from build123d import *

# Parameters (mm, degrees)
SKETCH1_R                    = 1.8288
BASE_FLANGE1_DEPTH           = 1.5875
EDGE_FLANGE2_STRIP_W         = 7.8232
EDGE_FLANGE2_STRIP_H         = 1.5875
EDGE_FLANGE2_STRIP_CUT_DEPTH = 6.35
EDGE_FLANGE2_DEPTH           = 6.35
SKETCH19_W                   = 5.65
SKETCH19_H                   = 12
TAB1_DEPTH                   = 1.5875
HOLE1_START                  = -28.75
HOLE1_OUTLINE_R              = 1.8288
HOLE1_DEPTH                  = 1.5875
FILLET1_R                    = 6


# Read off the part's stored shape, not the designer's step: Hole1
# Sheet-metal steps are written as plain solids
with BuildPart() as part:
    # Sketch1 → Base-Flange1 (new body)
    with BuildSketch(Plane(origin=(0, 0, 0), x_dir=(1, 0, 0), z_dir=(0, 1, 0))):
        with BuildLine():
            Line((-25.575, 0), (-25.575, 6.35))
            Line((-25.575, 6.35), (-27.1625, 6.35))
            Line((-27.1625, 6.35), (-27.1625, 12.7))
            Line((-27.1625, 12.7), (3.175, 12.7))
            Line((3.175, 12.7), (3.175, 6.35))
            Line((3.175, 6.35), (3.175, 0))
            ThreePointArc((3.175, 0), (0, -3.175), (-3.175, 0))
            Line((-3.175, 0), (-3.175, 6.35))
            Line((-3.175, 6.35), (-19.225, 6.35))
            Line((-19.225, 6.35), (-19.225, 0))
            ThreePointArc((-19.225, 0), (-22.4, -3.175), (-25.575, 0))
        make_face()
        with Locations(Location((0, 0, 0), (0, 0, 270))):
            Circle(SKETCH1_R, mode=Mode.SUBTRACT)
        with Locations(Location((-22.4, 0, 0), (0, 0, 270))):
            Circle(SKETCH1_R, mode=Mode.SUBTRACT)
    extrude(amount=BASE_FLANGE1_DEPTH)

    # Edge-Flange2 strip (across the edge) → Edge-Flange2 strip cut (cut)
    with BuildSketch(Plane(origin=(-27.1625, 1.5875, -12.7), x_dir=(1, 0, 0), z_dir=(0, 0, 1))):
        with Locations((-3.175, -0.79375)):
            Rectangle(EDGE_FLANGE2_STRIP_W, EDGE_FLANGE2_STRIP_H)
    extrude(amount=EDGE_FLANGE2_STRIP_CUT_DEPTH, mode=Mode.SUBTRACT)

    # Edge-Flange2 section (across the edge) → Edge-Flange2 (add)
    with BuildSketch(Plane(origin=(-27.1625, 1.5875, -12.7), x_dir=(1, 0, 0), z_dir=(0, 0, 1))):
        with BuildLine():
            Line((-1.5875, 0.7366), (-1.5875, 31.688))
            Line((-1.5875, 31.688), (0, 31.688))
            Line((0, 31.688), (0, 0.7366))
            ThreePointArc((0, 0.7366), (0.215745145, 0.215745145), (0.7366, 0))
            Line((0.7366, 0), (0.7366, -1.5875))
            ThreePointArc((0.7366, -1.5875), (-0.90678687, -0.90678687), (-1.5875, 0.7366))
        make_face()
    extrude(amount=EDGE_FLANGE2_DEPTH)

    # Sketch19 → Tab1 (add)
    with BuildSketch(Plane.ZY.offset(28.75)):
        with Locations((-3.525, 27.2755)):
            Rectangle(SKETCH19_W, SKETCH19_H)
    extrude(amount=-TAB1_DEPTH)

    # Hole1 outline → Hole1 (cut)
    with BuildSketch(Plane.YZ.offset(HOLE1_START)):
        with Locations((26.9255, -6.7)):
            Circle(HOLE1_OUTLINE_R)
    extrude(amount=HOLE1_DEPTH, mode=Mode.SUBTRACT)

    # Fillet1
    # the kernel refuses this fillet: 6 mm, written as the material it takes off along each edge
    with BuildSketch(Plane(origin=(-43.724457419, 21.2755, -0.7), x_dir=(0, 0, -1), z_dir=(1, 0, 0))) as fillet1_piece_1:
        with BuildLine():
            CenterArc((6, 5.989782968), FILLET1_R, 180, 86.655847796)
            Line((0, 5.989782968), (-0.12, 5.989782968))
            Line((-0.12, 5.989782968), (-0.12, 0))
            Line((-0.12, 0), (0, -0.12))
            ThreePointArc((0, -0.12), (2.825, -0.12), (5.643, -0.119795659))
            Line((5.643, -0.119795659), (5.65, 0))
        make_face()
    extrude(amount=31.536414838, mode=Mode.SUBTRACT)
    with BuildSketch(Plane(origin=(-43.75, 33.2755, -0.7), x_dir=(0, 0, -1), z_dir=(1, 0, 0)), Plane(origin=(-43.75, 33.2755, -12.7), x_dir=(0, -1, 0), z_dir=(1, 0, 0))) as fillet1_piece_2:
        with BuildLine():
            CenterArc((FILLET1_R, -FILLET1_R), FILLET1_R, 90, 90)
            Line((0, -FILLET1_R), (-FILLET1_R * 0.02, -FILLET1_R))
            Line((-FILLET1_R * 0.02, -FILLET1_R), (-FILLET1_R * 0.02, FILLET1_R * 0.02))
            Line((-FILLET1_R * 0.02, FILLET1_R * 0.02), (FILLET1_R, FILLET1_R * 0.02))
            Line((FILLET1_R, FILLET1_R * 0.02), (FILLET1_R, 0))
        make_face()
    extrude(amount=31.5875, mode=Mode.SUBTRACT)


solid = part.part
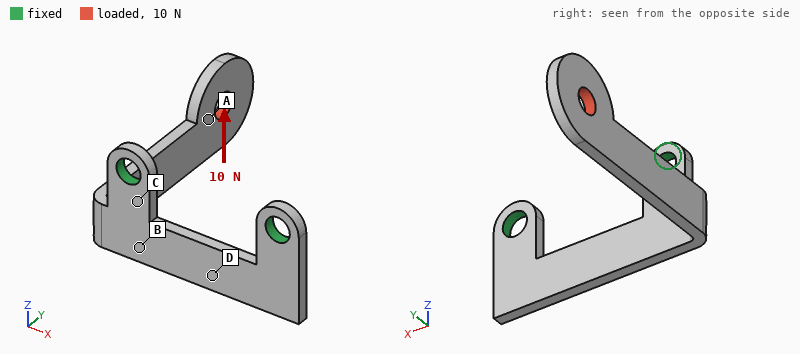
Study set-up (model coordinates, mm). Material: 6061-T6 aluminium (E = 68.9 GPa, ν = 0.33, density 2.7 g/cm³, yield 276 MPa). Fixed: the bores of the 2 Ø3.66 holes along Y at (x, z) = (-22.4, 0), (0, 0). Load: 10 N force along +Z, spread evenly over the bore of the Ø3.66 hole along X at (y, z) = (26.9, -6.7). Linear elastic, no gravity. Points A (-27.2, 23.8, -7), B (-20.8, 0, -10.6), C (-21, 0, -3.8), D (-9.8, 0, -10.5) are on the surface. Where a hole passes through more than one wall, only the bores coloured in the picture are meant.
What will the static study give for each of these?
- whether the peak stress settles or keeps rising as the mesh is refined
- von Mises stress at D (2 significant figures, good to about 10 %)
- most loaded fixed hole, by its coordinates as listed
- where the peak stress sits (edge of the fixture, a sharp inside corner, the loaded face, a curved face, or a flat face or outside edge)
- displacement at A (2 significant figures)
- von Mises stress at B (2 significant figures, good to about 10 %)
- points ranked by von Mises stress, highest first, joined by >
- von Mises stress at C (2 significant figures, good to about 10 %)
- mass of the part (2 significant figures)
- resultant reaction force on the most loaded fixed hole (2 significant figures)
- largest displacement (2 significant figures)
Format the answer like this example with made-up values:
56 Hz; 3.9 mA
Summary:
keeps rising; 21 MPa; (-22.4, 0); a sharp inside corner; 0.34 mm; 41 MPa; C > B > D > A; 71 MPa; 2.3 g; 12 N; 0.49 mm
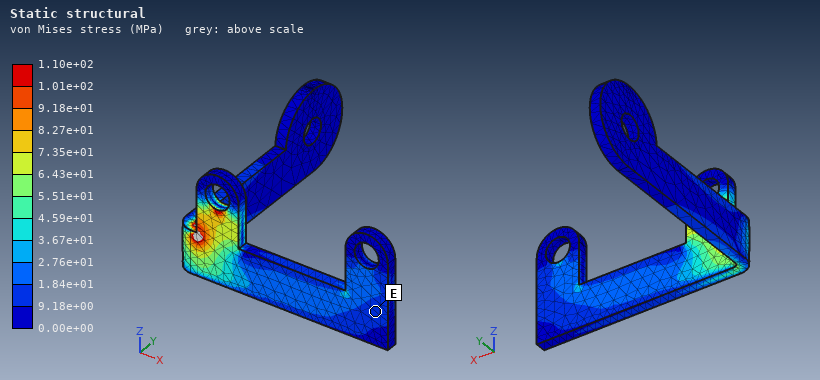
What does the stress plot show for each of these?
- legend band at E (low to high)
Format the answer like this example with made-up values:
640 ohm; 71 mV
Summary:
9.18e+00 to 1.84e+01 MPa
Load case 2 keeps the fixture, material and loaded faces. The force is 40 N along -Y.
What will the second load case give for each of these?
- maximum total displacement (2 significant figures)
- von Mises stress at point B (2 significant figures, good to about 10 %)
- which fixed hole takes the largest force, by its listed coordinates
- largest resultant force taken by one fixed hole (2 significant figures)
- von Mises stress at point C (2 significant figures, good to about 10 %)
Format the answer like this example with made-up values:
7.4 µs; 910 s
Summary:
0.24 mm; 26 MPa; (-22.4, 0); 43 N; 50 MPa
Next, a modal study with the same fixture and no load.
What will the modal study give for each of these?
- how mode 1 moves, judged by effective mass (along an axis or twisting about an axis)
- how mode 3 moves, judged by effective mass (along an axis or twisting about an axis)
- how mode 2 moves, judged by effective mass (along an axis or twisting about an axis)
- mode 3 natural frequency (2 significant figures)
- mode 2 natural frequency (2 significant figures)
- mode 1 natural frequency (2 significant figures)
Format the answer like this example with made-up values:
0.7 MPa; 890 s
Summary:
along X; along Y; along Z; 4700 Hz; 1000 Hz; 780 Hz
